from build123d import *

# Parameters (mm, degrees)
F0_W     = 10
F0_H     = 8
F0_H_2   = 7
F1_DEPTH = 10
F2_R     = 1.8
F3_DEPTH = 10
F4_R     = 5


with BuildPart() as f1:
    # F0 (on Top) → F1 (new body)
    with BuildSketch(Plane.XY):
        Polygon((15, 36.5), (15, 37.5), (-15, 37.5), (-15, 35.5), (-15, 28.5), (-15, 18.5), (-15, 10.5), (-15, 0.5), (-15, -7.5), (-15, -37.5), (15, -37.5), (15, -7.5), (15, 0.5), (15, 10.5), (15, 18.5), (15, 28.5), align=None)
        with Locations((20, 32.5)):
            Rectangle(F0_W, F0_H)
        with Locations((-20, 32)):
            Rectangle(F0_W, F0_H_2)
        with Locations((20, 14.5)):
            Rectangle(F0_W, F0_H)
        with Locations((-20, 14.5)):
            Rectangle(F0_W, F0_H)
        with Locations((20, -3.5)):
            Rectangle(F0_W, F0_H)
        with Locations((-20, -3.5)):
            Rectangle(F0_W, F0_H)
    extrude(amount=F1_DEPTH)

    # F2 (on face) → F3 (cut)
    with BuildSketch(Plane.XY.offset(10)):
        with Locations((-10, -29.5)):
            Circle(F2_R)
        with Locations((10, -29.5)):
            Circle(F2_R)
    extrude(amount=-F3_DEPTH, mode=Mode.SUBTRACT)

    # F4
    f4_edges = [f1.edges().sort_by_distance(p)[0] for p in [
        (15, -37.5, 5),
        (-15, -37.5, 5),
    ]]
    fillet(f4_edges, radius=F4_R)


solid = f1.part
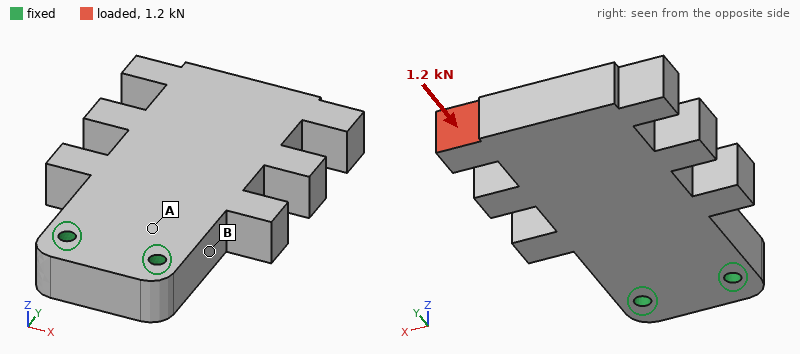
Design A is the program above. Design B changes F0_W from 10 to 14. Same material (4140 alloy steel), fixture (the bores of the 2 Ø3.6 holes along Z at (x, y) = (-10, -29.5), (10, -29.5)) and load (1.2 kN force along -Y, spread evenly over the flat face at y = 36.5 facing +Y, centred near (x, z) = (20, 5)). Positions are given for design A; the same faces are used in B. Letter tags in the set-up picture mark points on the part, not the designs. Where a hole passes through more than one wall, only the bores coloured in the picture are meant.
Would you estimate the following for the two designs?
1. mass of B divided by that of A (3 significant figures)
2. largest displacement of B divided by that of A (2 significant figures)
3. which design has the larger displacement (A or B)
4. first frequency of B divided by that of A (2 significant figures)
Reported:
1.03
1.2
B
0.98
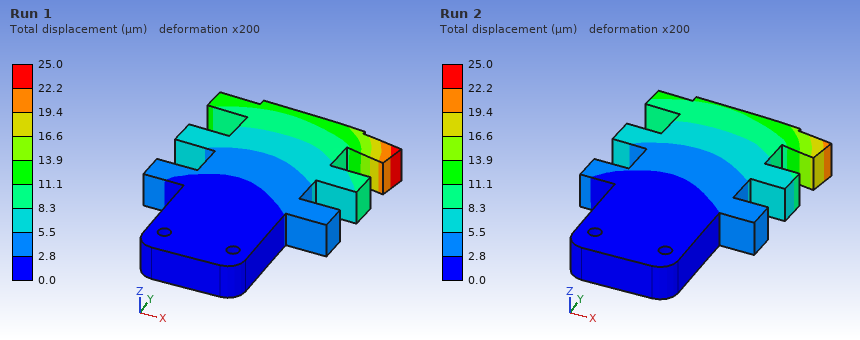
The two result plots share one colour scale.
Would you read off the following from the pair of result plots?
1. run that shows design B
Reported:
Run 1
